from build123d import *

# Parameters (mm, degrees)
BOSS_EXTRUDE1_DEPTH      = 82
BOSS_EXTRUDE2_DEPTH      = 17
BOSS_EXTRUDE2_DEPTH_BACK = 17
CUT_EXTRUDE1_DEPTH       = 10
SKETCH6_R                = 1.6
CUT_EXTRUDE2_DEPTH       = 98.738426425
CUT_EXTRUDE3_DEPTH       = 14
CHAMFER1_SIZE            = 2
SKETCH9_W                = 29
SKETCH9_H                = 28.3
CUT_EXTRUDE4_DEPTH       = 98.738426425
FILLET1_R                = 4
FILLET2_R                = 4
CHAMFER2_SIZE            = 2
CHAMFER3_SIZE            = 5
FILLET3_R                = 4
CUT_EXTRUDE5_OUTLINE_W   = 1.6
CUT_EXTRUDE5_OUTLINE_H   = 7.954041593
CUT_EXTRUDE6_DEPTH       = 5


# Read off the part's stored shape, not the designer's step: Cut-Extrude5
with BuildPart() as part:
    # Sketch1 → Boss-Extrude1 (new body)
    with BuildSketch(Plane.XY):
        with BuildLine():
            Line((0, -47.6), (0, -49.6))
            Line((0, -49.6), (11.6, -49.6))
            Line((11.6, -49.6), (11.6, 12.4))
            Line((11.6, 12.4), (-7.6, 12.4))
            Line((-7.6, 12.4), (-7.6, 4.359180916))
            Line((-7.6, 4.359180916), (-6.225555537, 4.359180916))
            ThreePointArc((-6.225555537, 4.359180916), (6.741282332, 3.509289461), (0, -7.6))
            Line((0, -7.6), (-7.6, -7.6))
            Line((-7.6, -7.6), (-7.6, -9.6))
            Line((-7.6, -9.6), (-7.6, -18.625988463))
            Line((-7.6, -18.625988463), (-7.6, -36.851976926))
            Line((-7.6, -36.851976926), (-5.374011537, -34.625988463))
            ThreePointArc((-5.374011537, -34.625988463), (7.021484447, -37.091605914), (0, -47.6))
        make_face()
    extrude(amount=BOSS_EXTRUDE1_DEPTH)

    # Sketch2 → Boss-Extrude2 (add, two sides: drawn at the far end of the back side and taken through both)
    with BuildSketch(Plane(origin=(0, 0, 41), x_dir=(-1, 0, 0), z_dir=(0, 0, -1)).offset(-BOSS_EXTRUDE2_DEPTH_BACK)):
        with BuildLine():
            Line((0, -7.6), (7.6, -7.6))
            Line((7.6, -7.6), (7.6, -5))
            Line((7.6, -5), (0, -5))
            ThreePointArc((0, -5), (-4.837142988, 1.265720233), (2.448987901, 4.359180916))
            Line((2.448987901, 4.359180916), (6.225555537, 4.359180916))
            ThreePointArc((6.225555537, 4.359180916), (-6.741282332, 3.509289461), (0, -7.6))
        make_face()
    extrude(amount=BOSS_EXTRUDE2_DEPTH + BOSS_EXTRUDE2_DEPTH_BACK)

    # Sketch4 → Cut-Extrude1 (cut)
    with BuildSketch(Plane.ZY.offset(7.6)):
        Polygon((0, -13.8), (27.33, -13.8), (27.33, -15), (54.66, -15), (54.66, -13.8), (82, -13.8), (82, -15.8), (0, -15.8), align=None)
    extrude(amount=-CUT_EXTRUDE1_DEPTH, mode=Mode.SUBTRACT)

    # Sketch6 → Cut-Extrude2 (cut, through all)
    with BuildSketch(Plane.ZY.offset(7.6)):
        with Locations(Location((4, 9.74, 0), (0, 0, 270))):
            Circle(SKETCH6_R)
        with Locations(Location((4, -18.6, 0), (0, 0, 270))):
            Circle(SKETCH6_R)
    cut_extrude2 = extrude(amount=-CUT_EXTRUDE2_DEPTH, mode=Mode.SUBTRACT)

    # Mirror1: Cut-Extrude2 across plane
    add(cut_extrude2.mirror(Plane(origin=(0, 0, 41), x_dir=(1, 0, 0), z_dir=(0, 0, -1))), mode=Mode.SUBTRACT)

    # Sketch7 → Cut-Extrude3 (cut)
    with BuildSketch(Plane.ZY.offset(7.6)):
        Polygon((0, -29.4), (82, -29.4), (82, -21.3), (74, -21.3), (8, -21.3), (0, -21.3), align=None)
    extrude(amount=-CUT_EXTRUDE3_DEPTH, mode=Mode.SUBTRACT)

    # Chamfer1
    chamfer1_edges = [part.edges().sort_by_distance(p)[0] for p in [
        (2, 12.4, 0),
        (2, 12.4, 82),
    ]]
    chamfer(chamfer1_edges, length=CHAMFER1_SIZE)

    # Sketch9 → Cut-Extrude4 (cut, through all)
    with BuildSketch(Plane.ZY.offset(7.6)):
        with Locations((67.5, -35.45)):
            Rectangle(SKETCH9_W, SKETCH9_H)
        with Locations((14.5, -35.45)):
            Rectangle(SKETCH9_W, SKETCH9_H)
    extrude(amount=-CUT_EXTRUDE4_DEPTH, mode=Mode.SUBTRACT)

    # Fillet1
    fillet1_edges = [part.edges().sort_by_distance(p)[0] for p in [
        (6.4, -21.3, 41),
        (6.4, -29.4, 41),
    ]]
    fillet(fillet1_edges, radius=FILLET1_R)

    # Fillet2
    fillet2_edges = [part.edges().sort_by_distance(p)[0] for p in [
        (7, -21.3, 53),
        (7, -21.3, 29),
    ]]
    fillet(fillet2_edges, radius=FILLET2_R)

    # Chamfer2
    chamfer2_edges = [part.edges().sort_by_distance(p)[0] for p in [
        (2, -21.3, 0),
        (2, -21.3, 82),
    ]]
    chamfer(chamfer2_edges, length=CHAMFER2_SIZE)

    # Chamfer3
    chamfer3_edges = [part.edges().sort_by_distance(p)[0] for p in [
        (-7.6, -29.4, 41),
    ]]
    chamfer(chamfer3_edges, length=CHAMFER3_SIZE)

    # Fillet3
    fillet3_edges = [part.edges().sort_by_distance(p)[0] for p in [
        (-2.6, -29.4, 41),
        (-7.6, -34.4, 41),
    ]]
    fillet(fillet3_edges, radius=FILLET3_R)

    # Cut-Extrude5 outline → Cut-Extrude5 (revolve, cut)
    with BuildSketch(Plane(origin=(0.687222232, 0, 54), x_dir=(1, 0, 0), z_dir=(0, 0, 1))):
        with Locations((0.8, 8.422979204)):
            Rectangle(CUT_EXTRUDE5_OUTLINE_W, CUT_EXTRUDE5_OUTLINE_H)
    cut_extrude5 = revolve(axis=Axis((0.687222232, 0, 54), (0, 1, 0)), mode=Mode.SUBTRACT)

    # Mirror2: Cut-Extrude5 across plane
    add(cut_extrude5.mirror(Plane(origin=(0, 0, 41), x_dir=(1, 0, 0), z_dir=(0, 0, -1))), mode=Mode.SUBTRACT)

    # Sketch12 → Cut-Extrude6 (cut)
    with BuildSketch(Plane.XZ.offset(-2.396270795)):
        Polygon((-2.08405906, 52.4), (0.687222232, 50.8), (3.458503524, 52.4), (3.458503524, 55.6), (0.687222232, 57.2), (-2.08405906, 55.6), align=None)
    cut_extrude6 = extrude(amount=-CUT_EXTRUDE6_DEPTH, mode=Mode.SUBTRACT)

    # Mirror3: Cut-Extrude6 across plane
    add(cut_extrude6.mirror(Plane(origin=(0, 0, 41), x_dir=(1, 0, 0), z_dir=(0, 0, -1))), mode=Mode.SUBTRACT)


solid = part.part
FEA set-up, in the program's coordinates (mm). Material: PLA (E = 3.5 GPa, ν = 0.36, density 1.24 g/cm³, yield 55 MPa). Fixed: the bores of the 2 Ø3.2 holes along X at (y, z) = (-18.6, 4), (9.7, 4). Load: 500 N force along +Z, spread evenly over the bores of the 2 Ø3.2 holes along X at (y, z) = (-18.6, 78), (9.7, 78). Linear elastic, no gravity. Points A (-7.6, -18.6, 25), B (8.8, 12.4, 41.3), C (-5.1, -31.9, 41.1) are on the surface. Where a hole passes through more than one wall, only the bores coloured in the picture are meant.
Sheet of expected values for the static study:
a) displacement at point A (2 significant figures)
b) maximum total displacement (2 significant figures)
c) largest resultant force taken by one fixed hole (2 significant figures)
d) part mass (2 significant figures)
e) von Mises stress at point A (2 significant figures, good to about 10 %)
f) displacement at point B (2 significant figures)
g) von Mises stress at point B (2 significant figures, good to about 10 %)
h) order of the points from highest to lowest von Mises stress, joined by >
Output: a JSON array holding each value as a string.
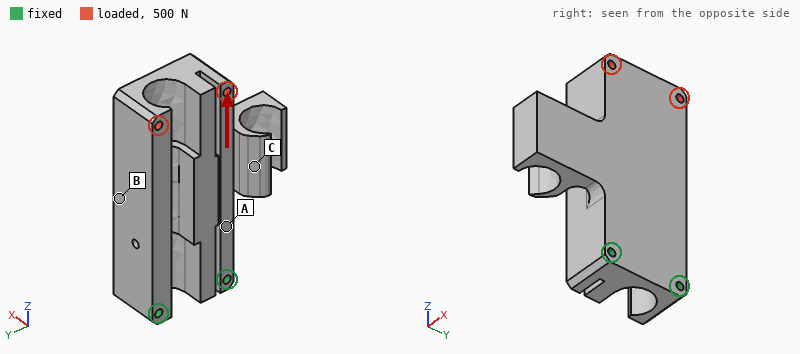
["14 µm", "70 µm", "260 N", "53 g", "1.7 MPa", "17 µm", "0.96 MPa", "A > B > C"]
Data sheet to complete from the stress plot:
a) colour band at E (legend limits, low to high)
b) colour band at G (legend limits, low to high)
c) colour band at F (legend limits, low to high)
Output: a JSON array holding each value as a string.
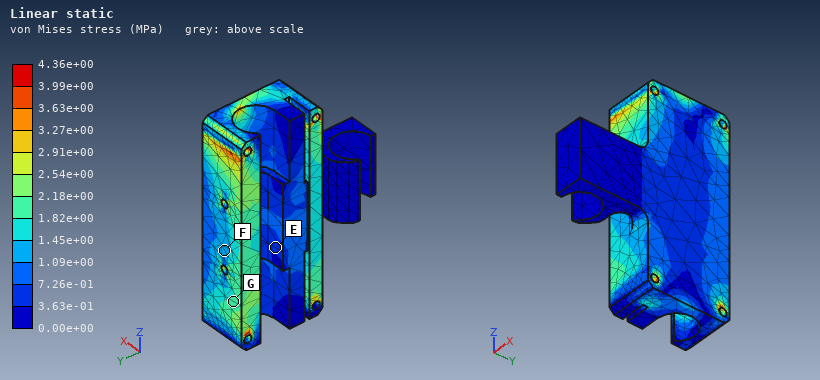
["3.63e-01 to 7.26e-01 MPa", "1.82e+00 to 2.18e+00 MPa", "1.09e+00 to 1.45e+00 MPa"]
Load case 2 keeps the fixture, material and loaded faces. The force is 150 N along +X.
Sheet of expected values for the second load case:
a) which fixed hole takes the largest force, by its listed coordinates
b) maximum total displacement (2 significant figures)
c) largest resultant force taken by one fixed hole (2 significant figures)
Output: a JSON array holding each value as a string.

["(9.7, 4)", "0.58 mm", "100 N"]
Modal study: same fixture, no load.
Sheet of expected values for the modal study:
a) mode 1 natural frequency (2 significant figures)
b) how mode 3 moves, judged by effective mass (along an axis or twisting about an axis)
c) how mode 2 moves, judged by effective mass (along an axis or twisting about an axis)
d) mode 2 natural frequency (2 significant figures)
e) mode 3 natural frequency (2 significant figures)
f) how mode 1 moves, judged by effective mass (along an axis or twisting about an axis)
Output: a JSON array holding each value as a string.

["690 Hz", "along Y", "along Y", "950 Hz", "1300 Hz", "along X"]
